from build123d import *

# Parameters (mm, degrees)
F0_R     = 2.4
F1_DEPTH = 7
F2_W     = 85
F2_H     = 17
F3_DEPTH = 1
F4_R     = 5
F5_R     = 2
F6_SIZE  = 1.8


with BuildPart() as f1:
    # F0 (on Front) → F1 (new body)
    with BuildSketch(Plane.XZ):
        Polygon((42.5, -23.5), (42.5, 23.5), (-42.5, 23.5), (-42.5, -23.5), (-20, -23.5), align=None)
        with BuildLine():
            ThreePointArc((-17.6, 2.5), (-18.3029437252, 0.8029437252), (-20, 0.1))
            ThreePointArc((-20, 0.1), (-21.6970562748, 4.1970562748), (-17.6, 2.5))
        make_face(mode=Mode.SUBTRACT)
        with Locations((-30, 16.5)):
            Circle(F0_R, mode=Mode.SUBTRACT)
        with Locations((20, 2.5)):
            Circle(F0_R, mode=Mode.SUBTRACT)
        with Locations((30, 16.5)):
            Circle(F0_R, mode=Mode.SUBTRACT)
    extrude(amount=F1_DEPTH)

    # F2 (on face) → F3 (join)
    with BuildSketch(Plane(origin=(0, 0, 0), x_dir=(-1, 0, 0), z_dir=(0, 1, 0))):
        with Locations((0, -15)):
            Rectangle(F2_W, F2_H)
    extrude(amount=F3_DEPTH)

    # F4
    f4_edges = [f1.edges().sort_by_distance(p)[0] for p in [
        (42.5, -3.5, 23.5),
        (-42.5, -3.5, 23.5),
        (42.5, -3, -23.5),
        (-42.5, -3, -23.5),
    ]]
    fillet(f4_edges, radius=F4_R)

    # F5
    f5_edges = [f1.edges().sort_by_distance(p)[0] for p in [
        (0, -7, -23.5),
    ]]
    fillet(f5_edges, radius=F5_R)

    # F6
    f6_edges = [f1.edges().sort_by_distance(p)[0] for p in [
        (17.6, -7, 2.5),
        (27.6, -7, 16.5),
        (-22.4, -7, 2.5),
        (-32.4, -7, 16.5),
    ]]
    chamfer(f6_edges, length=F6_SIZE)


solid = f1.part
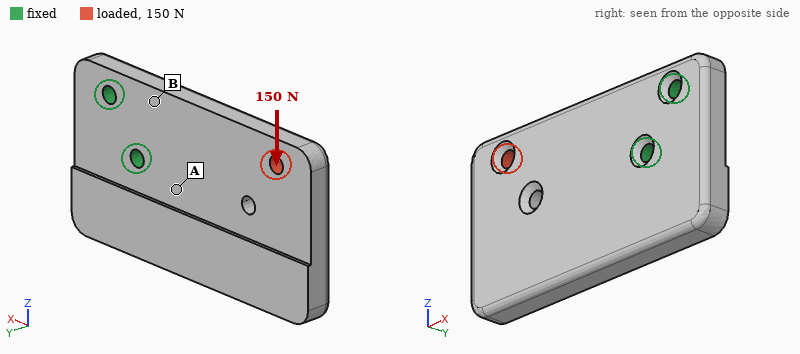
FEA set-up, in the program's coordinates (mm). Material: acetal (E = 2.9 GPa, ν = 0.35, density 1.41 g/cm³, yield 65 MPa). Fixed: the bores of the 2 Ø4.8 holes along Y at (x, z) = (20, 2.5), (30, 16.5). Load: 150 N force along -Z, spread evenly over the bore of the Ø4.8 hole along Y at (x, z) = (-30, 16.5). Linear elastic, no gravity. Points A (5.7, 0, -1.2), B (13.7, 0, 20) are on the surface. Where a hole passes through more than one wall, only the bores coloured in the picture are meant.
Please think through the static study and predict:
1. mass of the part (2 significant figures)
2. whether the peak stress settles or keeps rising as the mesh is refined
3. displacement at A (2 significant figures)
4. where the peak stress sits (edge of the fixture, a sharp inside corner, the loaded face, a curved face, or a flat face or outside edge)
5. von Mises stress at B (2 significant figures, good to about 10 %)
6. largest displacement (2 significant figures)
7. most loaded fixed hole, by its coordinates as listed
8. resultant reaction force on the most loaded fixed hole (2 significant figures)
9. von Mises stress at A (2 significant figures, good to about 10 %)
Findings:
40 g
keeps rising
0.045 mm
edge of the fixture
3.4 MPa
0.22 mm
(20, 2.5)
450 N
1.3 MPa
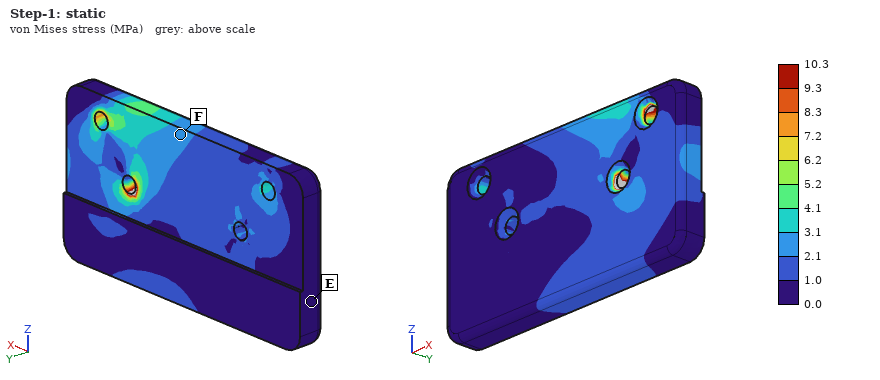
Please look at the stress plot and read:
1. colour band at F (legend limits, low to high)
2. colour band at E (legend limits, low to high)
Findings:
2.1 to 3.1 MPa
0.0 to 1.0 MPa
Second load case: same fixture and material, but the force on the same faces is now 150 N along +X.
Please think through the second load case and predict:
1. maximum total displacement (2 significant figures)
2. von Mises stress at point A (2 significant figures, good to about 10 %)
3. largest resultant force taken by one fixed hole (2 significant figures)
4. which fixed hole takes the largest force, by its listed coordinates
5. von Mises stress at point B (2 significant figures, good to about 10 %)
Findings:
95 µm
0.70 MPa
120 N
(30, 16.5)
1.6 MPa
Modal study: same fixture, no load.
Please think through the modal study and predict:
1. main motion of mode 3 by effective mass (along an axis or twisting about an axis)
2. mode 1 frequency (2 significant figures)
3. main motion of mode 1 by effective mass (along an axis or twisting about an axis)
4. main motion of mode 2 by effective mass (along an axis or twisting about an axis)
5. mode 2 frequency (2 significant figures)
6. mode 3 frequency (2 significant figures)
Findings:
along Z
370 Hz
along Y
twisting about X
930 Hz
1200 Hz
